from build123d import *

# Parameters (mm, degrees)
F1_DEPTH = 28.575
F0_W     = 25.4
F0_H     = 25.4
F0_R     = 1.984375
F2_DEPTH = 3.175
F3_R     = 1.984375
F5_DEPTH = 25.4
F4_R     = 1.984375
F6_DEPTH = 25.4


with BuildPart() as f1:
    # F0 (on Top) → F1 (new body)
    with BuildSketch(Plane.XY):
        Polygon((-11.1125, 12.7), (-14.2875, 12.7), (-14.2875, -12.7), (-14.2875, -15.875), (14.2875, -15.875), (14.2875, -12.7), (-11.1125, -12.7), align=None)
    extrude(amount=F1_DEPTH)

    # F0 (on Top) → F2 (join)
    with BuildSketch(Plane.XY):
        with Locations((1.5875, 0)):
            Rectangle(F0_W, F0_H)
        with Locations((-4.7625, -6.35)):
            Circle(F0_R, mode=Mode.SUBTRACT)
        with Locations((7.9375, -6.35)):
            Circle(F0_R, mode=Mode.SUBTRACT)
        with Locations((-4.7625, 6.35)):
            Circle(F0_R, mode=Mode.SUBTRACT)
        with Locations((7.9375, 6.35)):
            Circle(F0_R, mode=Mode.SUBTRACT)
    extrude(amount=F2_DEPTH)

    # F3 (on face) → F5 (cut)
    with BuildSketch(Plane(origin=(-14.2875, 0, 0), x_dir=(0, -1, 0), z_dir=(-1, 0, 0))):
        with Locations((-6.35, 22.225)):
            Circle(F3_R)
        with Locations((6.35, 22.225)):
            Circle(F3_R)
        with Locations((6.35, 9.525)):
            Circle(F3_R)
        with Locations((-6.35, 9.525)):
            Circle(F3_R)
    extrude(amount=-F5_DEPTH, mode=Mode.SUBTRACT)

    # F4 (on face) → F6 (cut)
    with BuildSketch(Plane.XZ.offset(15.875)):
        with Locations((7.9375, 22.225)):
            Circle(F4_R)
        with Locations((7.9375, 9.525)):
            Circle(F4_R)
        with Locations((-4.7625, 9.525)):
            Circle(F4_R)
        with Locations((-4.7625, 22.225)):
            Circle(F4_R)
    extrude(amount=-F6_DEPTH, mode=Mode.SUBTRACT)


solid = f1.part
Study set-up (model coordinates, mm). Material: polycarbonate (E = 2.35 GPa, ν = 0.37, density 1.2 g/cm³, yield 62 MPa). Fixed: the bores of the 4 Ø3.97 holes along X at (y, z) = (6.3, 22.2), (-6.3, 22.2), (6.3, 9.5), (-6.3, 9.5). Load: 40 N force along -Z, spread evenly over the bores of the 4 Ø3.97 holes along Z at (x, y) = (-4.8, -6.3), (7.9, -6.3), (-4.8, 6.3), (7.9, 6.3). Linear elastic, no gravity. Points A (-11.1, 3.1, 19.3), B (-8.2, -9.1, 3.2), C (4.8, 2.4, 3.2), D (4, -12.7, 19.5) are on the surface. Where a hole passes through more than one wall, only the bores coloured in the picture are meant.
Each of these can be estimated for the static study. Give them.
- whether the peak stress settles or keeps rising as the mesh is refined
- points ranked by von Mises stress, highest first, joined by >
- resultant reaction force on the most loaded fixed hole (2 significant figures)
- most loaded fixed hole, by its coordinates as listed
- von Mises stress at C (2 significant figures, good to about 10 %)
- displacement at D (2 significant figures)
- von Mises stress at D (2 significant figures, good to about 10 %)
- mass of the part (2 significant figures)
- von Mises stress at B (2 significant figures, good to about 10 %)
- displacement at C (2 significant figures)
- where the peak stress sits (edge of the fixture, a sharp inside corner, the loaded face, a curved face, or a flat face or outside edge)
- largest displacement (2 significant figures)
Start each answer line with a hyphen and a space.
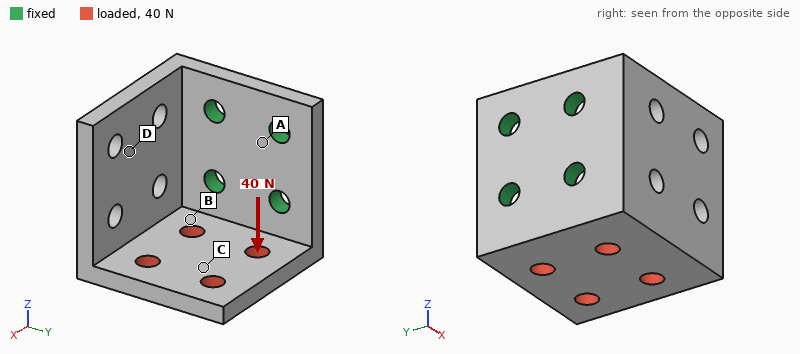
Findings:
- keeps rising
- C > B > D > A
- 33 N
- (-6.3, 9.5)
- 3.1 MPa
- 0.11 mm
- 1.0 MPa
- 7.8 g
- 2.4 MPa
- 0.23 mm
- edge of the fixture
- 0.49 mm
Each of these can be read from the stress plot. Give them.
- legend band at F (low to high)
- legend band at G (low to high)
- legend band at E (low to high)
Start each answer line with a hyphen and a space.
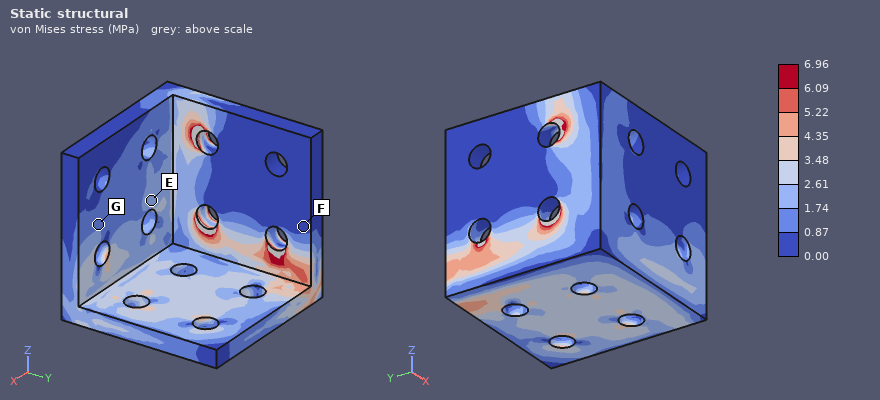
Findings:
- 0.00 to 0.87 MPa
- 0.87 to 1.74 MPa
- 1.74 to 2.61 MPa
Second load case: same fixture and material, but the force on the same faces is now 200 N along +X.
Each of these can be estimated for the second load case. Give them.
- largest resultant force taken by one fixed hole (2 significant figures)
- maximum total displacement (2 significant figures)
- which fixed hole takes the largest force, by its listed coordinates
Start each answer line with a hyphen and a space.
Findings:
- 130 N
- 0.42 mm
- (-6.3, 9.5)
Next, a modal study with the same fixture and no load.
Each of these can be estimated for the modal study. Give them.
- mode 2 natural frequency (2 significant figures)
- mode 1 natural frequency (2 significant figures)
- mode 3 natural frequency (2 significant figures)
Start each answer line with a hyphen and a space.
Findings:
- 1400 Hz
- 1100 Hz
- 2000 Hz
